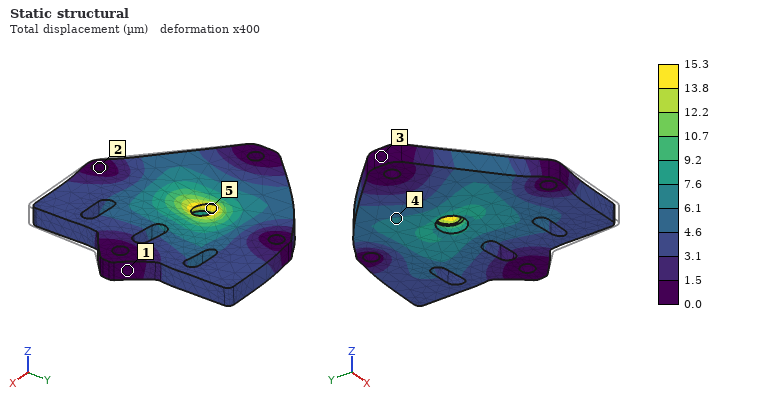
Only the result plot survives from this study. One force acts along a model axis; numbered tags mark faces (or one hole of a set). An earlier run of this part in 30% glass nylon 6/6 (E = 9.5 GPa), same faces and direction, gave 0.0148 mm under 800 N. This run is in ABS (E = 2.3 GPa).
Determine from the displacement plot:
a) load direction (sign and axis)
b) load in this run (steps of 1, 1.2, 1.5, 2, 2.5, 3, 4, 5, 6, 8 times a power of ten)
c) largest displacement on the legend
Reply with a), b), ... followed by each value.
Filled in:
a) +Y
b) 200 N
c) 15.3 µm
